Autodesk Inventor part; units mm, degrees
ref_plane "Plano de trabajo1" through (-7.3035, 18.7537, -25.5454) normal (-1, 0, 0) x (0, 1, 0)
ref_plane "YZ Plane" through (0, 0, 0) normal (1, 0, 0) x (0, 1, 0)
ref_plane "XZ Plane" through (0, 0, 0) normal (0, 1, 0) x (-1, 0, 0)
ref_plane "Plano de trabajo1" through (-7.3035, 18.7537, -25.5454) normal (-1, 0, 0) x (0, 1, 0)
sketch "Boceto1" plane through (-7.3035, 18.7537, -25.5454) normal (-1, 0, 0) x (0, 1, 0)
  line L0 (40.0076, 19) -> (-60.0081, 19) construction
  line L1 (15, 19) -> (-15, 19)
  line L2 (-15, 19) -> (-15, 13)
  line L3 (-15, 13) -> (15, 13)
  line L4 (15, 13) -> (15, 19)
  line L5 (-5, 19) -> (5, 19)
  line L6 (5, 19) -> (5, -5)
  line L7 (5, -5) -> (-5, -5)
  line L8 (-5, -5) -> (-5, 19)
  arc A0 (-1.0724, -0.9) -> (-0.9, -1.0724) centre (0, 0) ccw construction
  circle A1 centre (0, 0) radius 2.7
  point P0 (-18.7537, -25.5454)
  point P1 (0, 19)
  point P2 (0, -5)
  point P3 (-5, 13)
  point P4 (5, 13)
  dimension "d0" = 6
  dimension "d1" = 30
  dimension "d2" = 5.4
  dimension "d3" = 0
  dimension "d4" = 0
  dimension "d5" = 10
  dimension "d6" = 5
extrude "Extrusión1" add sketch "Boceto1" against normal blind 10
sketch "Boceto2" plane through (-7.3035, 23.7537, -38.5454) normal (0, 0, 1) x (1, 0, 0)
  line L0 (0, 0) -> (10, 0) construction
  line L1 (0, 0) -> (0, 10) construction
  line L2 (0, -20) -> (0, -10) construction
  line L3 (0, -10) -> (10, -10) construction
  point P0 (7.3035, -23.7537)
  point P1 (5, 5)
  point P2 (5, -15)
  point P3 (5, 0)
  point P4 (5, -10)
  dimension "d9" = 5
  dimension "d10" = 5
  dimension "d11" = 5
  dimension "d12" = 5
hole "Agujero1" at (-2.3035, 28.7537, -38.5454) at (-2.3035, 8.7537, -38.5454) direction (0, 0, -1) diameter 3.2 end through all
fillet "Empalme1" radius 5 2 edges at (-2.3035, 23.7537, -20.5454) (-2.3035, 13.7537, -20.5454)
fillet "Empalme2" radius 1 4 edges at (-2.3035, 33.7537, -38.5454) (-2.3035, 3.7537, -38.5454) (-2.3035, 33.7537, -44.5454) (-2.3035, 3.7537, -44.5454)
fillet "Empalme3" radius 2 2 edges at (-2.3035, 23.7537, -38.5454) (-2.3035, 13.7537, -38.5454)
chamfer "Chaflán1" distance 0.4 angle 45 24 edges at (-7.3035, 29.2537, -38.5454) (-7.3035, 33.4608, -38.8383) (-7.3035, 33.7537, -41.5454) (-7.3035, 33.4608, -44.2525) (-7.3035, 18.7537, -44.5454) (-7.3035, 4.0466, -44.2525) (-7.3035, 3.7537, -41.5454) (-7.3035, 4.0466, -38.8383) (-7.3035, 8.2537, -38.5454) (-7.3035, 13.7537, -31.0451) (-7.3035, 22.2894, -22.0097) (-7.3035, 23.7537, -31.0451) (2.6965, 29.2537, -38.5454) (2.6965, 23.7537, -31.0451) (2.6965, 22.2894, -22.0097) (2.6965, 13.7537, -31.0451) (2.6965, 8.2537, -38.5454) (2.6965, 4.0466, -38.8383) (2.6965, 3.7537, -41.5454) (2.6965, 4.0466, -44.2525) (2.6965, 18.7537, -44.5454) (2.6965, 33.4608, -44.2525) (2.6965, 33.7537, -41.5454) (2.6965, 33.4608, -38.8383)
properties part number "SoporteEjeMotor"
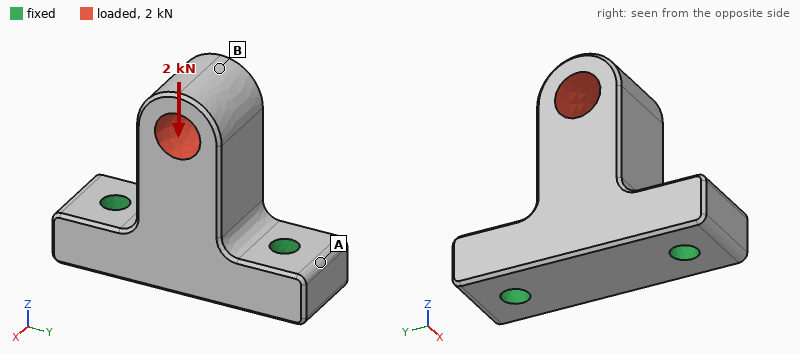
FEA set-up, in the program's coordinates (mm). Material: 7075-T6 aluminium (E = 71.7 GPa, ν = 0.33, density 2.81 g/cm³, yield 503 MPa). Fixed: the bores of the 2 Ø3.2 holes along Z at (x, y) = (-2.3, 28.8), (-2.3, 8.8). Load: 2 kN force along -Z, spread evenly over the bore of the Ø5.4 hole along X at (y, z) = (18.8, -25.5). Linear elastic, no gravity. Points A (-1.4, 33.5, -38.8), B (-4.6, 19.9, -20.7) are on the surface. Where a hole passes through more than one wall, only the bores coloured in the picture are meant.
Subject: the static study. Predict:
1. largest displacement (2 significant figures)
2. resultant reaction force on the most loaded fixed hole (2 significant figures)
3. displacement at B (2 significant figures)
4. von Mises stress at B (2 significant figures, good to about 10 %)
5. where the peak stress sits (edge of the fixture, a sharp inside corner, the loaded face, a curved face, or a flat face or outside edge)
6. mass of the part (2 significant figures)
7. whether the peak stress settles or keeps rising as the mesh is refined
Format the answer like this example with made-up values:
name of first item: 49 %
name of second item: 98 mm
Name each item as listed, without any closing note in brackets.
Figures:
largest displacement: 13 µm
resultant reaction force on the most loaded fixed hole: 1.1 kN
displacement at B: 12 µm
von Mises stress at B: 26 MPa
where the peak stress sits: edge of the fixture
mass of the part: 8.9 g
whether the peak stress settles or keeps rising as the mesh is refined: keeps rising
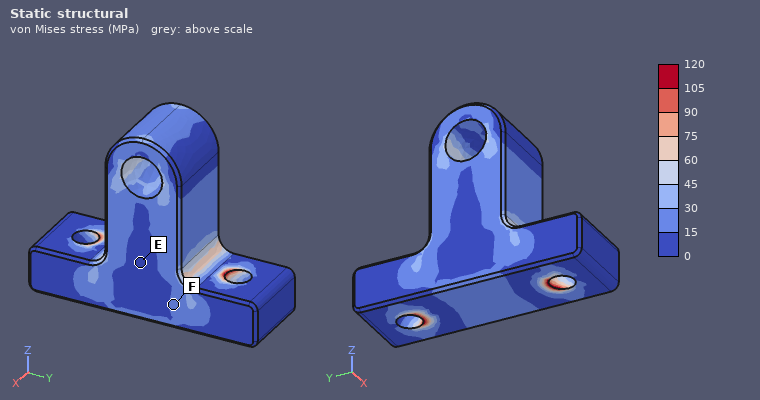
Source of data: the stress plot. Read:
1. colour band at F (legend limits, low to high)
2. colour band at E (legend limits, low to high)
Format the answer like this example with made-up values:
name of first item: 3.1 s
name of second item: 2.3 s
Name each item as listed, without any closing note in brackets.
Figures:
colour band at F: 15 to 30 MPa
colour band at E: 0 to 15 MPa
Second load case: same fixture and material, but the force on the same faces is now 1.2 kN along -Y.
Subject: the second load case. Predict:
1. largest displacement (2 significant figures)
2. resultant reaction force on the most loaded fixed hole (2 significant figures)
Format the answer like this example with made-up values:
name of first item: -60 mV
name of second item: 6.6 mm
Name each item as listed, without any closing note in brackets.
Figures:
largest displacement: 54 µm
resultant reaction force on the most loaded fixed hole: 1.3 kN
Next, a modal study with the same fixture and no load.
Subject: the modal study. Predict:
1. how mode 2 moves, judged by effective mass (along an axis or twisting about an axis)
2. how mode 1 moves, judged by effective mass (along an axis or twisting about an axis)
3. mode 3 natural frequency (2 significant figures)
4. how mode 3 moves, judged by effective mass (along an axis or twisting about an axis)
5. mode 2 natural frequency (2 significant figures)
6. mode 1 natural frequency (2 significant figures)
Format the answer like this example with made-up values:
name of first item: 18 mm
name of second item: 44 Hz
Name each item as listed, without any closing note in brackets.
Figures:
how mode 2 moves, judged by effective mass: along Y
how mode 1 moves, judged by effective mass: along X
mode 3 natural frequency: 36 kHz
how mode 3 moves, judged by effective mass: along Z
mode 2 natural frequency: 20 kHz
mode 1 natural frequency: 12 kHz
